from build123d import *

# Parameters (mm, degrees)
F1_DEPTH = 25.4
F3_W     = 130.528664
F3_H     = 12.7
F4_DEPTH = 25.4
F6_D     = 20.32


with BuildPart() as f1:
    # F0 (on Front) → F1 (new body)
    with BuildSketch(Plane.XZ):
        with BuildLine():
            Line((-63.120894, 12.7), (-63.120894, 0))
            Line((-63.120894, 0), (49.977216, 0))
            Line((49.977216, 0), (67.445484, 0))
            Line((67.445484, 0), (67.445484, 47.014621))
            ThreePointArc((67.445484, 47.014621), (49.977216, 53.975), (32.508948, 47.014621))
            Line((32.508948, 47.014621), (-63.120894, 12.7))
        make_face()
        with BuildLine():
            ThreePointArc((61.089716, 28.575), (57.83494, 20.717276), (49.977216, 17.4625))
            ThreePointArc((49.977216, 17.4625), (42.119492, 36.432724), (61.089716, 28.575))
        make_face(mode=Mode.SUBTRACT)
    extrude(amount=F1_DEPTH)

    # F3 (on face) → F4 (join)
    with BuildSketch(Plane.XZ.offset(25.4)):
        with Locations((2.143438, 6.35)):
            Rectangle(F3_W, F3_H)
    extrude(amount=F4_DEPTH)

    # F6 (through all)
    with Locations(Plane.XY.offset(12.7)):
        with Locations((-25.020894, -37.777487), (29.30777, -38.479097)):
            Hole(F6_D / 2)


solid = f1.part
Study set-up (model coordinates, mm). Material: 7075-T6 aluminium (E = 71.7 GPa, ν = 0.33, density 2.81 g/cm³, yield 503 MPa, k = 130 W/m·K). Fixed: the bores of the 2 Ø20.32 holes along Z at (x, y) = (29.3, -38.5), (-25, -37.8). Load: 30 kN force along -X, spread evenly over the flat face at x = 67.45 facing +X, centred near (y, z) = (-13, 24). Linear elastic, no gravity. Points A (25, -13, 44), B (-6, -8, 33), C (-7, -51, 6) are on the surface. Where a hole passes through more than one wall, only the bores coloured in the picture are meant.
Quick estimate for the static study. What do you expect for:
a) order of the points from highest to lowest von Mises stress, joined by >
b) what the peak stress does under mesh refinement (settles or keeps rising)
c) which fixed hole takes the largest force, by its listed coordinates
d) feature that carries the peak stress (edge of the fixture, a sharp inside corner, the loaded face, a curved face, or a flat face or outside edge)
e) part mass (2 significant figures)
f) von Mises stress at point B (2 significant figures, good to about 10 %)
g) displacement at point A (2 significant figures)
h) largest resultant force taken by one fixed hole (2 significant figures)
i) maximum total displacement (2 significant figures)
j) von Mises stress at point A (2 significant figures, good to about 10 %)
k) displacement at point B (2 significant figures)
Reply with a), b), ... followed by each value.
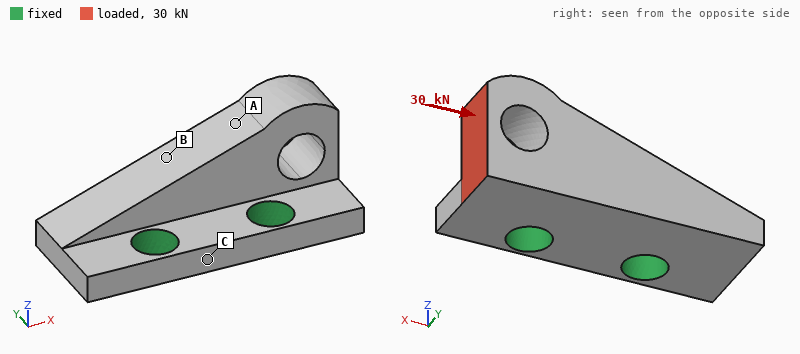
a) A > B > C
b) keeps rising
c) (29.3, -38.5)
d) edge of the fixture
e) 400 g
f) 34 MPa
g) 0.060 mm
h) 20 kN
i) 0.12 mm
j) 59 MPa
k) 0.031 mm
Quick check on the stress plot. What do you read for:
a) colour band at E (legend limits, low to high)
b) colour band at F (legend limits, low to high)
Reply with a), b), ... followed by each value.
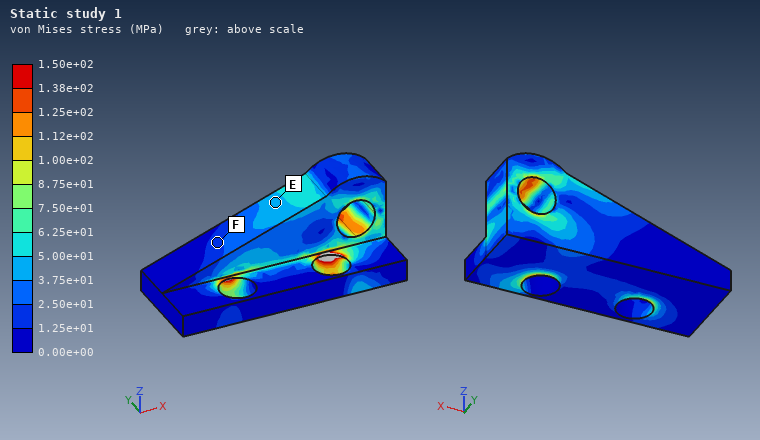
a) 3.75e+01 to 5.00e+01 MPa
b) 1.25e+01 to 2.50e+01 MPa
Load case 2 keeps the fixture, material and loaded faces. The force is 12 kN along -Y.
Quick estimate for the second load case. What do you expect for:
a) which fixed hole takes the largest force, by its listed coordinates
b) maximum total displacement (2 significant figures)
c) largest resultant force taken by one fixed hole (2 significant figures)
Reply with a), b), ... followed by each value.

a) (29.3, -38.5)
b) 0.24 mm
c) 17 kN
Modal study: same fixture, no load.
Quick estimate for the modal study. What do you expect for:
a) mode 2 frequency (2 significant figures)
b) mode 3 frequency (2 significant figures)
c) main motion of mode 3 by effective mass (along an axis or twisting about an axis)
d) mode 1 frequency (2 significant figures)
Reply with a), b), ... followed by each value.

a) 6100 Hz
b) 8000 Hz
c) along Z
d) 3400 Hz
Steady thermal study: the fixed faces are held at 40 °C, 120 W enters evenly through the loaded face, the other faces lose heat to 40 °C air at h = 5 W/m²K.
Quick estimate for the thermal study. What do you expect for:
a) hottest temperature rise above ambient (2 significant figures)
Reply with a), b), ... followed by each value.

a) 53 K
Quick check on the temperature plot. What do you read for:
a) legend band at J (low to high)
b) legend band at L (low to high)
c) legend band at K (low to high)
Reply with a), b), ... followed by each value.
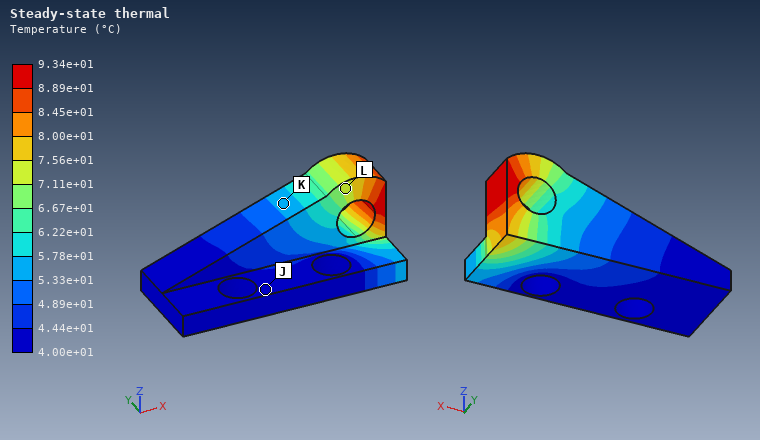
a) 4.00e+01 to 4.44e+01 °C
b) 7.11e+01 to 7.56e+01 °C
c) 5.33e+01 to 5.78e+01 °C
